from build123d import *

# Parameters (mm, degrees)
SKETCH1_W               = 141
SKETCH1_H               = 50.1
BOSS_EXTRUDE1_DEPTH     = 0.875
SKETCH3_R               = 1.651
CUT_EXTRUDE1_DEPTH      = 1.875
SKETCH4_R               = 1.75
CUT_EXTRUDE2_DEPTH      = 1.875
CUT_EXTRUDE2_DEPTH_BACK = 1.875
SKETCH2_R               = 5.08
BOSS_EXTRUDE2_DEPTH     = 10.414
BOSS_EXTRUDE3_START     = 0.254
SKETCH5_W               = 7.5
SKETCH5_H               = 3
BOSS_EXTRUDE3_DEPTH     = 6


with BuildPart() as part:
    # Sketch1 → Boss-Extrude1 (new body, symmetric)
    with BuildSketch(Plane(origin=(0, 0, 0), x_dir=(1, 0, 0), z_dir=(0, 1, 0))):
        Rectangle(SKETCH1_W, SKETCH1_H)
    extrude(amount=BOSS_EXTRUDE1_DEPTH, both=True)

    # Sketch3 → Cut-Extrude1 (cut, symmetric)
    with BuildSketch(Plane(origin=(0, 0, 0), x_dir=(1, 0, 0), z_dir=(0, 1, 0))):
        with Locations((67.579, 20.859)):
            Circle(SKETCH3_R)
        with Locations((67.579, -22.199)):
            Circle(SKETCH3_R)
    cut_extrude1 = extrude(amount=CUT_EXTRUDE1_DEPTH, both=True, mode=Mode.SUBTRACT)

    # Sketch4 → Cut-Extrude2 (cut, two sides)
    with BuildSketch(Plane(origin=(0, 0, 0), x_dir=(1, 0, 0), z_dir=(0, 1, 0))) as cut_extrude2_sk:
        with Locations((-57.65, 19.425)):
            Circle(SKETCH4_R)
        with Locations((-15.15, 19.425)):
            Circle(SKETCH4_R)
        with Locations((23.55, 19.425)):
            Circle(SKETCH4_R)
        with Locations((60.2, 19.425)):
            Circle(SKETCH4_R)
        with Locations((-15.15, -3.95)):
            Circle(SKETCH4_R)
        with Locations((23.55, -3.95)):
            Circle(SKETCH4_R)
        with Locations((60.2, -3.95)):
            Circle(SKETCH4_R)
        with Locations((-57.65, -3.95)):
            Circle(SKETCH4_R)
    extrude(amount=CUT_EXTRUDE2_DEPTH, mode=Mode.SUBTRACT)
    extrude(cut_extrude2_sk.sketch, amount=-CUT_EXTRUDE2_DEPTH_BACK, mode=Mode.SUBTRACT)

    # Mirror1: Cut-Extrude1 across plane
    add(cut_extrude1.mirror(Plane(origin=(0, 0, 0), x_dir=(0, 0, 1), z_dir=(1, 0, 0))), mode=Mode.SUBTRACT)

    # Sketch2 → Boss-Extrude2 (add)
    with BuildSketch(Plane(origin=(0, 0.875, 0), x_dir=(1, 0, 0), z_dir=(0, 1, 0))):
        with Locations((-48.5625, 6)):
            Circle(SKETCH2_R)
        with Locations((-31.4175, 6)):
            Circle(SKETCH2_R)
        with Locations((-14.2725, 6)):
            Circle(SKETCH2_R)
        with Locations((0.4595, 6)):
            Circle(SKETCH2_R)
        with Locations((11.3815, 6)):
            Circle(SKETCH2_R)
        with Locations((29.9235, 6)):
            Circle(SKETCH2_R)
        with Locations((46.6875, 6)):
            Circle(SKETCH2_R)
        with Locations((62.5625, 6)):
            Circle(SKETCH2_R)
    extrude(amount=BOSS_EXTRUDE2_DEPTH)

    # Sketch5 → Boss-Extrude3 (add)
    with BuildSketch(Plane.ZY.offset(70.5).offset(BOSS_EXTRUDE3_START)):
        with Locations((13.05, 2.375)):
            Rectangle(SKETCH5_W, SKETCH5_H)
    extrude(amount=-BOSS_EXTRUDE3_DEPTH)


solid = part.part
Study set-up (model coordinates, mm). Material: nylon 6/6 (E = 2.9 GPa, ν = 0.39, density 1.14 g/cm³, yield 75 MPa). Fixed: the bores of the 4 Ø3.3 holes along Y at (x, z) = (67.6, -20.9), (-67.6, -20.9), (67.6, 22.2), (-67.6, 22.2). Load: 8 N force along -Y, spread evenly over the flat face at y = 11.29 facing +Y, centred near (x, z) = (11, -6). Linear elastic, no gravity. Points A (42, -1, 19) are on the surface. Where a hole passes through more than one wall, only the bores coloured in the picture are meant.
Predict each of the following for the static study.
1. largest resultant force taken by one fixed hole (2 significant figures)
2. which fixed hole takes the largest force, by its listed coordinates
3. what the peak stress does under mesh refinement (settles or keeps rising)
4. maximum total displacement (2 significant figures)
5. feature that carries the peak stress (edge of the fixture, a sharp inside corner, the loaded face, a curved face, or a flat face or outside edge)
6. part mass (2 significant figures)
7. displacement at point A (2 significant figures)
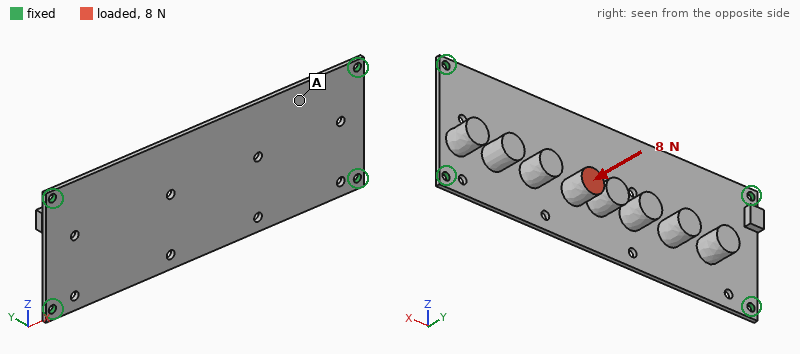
3.5 N
(67.6, -20.9)
keeps rising
1.6 mm
edge of the fixture
22 g
0.56 mm
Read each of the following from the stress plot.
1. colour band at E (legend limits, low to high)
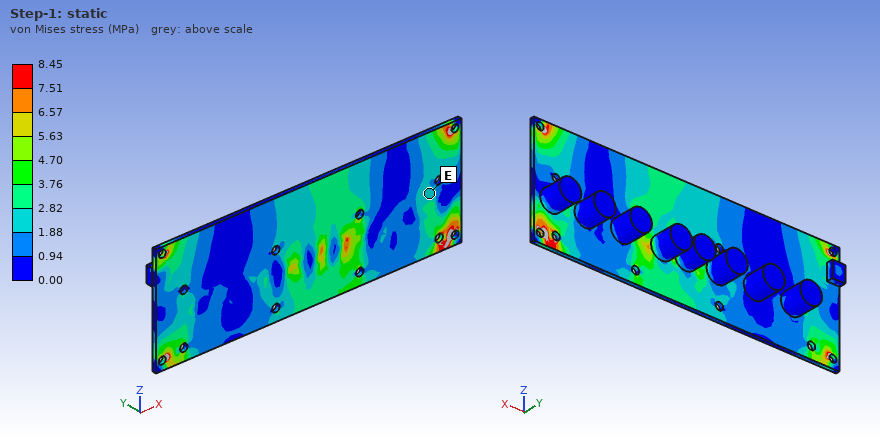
1.88 to 2.82 MPa
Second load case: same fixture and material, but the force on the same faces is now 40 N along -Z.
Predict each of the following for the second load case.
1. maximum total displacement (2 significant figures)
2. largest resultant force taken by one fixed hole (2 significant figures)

1.8 mm
21 N
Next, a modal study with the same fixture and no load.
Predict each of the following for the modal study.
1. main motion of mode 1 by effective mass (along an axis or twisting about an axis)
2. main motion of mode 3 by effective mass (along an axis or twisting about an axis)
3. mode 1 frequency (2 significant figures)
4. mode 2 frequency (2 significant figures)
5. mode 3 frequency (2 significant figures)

along Y
twisting about Z
120 Hz
330 Hz
340 Hz
